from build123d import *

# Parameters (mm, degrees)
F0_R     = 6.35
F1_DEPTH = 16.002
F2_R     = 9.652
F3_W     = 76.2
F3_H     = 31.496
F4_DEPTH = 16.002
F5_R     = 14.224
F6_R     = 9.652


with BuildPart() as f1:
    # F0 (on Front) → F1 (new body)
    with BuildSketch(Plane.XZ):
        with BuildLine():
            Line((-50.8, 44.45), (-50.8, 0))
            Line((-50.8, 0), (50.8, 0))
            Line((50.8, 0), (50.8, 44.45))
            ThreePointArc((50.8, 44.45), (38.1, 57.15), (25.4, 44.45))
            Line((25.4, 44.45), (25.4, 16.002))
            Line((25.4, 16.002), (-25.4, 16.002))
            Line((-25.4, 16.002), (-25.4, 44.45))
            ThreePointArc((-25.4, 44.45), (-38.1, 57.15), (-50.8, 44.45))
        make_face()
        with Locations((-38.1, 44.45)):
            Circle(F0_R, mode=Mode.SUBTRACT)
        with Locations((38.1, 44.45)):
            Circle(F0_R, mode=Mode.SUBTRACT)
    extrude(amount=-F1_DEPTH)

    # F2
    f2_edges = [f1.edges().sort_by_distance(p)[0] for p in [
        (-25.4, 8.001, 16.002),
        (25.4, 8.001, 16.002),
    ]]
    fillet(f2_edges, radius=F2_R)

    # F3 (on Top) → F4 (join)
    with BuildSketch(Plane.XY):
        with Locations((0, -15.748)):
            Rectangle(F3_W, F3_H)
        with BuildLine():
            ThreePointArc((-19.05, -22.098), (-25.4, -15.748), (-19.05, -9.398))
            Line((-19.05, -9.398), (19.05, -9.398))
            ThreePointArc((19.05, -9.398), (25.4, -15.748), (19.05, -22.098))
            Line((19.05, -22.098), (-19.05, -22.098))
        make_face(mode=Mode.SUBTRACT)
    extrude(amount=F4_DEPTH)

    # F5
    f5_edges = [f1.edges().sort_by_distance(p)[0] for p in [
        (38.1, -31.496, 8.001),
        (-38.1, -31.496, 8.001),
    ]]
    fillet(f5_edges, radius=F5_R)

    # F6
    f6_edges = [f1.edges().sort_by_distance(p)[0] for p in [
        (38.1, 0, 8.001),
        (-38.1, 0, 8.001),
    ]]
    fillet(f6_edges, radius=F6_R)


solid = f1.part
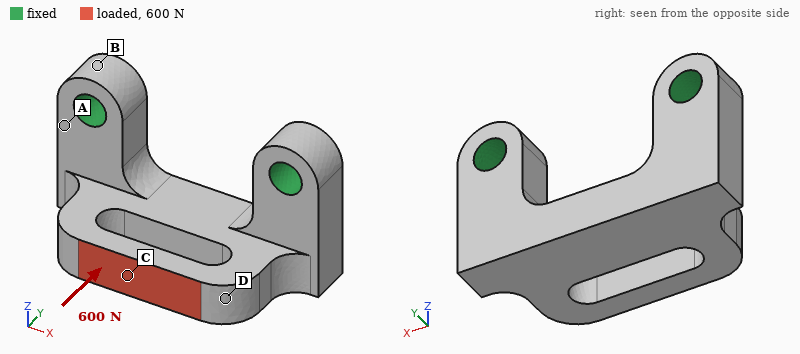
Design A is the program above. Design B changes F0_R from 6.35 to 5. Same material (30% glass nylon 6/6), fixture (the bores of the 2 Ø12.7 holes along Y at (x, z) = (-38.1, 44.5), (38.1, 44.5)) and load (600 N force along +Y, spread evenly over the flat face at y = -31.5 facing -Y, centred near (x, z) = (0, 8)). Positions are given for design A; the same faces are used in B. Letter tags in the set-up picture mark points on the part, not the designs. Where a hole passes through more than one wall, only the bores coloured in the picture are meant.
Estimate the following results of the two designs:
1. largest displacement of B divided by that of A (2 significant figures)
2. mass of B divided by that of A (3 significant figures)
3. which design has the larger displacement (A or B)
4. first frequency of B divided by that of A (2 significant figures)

1.1
1.02
B
0.95
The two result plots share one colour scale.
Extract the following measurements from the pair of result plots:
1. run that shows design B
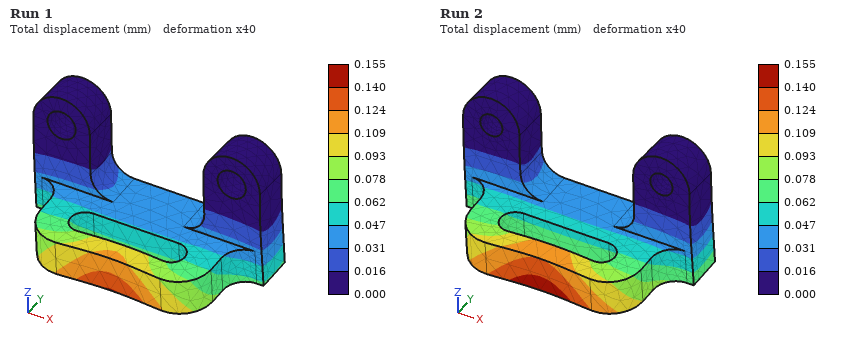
Run 2
